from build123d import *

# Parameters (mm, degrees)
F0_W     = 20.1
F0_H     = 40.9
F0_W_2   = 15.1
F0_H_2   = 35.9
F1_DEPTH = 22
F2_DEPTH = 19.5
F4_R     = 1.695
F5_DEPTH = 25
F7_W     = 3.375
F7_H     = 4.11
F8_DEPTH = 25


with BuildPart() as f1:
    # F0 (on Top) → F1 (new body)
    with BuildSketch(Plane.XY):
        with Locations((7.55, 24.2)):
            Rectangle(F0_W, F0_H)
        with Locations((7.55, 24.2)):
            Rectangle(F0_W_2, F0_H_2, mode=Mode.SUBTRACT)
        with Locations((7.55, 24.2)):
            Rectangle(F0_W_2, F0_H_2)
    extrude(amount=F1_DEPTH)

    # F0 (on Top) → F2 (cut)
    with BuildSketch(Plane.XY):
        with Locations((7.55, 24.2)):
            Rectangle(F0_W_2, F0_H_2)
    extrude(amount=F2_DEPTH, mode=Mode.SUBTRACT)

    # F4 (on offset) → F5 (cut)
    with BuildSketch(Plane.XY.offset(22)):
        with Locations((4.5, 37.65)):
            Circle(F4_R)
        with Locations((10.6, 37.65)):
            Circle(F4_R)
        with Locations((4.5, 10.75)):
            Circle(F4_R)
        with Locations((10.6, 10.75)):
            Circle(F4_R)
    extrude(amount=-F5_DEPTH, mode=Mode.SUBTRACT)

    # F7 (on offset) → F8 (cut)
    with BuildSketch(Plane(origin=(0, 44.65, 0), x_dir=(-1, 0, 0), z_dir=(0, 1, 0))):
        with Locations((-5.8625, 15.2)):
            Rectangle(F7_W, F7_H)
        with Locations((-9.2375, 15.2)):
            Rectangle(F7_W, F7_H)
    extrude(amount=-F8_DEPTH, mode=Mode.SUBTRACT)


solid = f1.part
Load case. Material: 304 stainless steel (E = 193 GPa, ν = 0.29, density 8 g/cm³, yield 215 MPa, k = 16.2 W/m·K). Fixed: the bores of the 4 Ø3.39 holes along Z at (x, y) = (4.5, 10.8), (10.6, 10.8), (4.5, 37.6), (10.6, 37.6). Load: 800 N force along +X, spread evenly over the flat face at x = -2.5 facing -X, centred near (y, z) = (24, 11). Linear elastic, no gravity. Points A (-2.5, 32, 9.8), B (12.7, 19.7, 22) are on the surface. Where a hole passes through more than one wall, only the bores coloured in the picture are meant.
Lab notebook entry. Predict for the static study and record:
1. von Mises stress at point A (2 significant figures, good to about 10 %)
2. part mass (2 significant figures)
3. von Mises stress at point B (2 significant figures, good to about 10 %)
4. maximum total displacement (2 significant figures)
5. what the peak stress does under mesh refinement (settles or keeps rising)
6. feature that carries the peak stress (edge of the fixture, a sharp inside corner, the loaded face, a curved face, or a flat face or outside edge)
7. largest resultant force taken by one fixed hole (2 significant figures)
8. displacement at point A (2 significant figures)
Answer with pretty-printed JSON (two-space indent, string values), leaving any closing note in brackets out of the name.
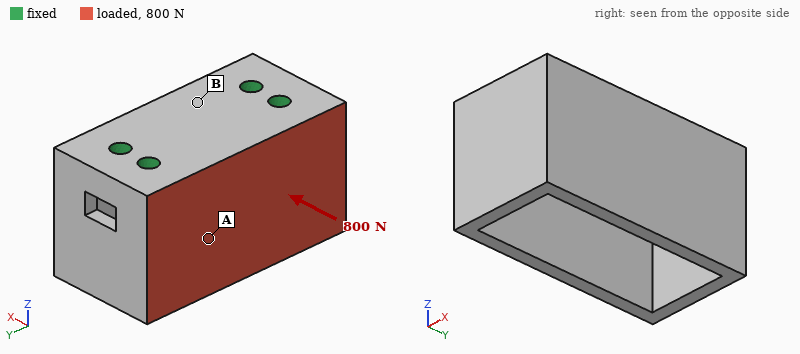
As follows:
{
  "von Mises stress at point A": "30 MPa",
  "part mass": "59 g",
  "von Mises stress at point B": "12 MPa",
  "maximum total displacement": "35 µm",
  "what the peak stress does under mesh refinement": "keeps rising",
  "feature that carries the peak stress": "edge of the fixture",
  "largest resultant force taken by one fixed hole": "430 N",
  "displacement at point A": "17 µm"
}
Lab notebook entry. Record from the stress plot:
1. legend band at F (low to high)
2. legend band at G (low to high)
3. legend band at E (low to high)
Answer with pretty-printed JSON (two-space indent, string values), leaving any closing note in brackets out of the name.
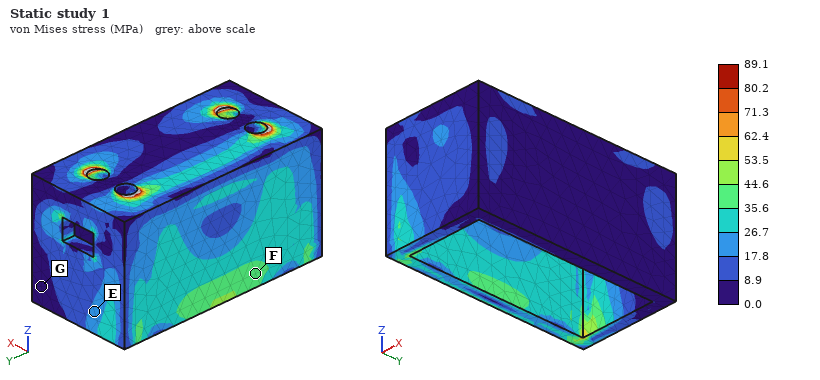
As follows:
{
  "legend band at F": "35.6 to 44.6 MPa",
  "legend band at G": "0.0 to 8.9 MPa",
  "legend band at E": "17.8 to 26.7 MPa"
}
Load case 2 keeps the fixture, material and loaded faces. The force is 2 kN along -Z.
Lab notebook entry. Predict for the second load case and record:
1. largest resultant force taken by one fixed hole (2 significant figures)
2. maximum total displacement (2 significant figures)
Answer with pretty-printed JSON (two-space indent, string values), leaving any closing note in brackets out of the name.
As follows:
{
  "largest resultant force taken by one fixed hole": "1.4 kN",
  "maximum total displacement": "36 µm"
}
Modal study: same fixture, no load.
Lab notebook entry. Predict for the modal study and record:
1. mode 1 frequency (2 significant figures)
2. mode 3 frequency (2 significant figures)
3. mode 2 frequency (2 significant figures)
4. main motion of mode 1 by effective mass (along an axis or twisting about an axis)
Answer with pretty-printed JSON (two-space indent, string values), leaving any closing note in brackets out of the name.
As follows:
{
  "mode 1 frequency": "6100 Hz",
  "mode 3 frequency": "8500 Hz",
  "mode 2 frequency": "7900 Hz",
  "main motion of mode 1 by effective mass": "along X"
}
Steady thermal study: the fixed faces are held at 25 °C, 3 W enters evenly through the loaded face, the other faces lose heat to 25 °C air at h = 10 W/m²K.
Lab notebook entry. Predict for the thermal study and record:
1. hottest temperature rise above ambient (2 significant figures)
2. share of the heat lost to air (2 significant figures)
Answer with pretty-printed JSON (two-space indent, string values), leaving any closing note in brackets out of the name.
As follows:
{
  "hottest temperature rise above ambient": "20 K",
  "share of the heat lost to air": "12 %"
}
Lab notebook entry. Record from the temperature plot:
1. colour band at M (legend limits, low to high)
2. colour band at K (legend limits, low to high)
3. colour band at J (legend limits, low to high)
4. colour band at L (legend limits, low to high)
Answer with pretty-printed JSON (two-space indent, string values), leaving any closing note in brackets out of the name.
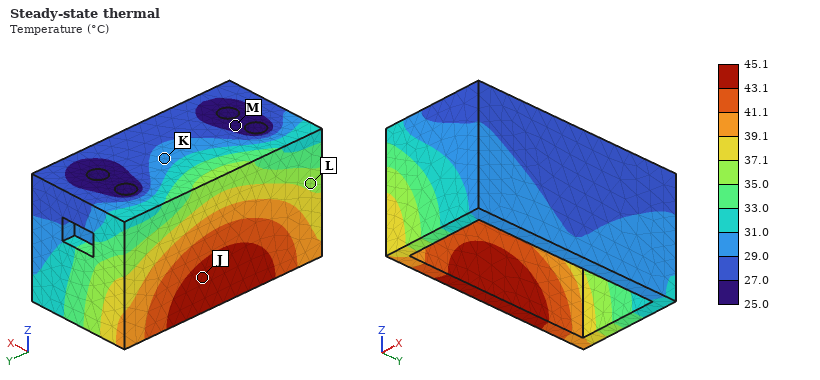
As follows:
{
  "colour band at M": "25.0 to 27.0 °C",
  "colour band at K": "29.0 to 31.0 °C",
  "colour band at J": "43.1 to 45.1 °C",
  "colour band at L": "35.0 to 37.1 °C"
}
